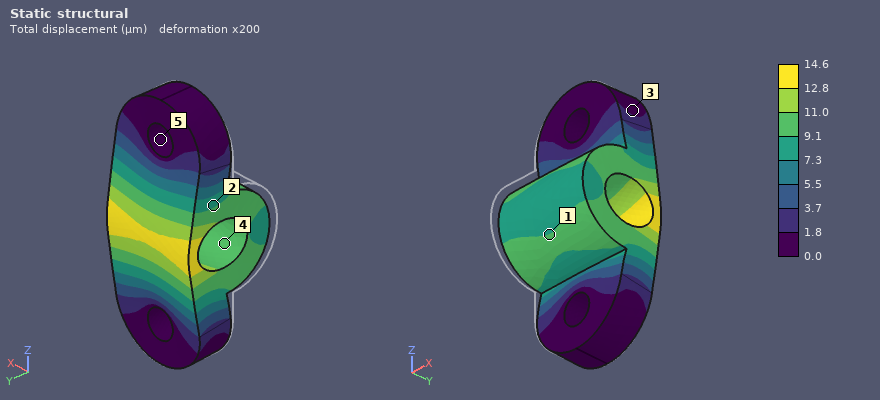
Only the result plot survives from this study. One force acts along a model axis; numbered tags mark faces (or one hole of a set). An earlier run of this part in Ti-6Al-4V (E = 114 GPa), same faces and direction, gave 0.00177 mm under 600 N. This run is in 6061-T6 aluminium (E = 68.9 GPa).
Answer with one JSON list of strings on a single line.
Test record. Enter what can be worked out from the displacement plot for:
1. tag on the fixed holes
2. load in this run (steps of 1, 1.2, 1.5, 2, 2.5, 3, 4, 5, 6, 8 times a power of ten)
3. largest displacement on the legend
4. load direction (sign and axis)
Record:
["5", "3 kN", "14.6 µm", "+Y"]
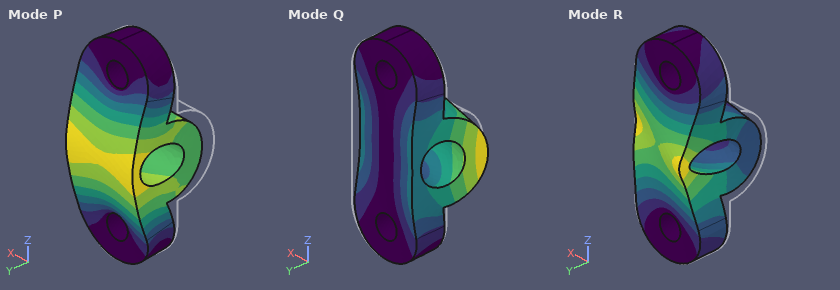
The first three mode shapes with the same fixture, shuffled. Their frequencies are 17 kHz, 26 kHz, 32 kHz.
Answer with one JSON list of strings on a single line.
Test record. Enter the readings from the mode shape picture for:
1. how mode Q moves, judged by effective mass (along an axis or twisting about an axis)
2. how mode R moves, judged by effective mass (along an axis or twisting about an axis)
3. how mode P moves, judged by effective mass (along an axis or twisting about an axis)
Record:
["along X", "along X", "along Y"]
